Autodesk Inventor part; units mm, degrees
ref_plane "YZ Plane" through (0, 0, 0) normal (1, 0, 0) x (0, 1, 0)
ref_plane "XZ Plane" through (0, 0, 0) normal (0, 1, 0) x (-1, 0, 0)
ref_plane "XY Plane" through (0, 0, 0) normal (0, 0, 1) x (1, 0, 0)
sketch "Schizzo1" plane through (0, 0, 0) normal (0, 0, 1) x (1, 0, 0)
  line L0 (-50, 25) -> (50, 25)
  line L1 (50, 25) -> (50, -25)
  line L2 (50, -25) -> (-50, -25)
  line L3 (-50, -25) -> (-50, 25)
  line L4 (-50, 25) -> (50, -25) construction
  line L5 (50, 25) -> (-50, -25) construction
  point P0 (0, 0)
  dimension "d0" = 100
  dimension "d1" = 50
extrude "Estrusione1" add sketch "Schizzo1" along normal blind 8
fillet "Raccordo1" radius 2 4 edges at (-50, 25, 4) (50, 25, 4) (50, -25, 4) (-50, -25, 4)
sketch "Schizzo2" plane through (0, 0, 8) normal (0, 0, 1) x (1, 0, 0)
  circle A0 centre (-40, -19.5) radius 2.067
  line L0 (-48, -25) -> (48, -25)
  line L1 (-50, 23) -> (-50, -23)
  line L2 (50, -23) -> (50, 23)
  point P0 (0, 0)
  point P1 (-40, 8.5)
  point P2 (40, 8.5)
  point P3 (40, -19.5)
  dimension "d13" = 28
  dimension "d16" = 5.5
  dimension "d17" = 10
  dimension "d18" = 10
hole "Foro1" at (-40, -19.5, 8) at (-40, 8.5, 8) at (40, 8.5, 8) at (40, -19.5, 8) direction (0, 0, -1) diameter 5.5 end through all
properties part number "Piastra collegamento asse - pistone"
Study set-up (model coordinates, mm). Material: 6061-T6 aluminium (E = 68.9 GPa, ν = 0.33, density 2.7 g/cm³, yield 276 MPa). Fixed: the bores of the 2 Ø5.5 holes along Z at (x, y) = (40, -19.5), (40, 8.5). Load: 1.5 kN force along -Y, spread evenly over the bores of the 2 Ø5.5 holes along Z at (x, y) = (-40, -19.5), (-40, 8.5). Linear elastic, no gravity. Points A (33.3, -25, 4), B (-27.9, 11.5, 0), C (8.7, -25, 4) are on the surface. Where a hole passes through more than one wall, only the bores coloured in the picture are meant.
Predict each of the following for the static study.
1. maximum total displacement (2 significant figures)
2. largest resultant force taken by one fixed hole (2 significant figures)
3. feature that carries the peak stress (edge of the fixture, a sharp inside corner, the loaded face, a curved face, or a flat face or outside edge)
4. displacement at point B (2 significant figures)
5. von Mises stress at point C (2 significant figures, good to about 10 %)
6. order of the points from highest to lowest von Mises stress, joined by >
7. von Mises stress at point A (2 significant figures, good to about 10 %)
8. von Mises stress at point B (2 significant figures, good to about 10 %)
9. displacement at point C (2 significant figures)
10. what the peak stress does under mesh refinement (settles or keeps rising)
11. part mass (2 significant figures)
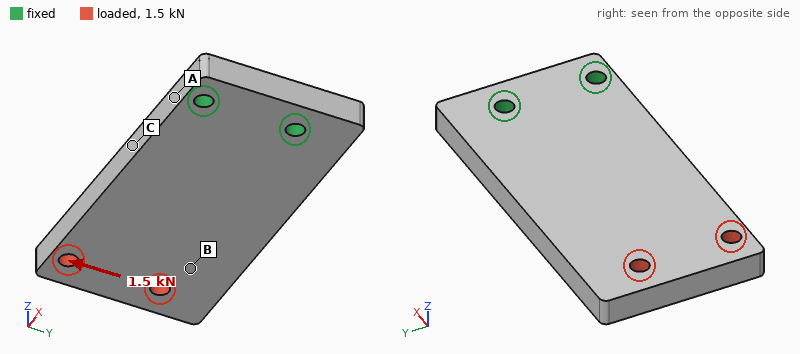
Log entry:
88 µm
4.0 kN
edge of the fixture
60 µm
23 MPa
A > C > B
39 MPa
8.1 MPa
26 µm
keeps rising
110 g
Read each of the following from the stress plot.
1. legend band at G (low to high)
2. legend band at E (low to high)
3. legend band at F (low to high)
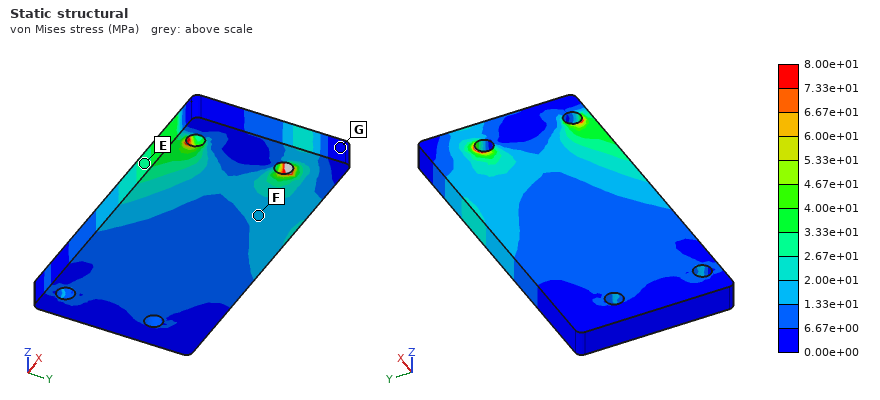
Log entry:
0.00e+00 to 6.67e+00 MPa
2.67e+01 to 3.33e+01 MPa
1.33e+01 to 2.00e+01 MPa
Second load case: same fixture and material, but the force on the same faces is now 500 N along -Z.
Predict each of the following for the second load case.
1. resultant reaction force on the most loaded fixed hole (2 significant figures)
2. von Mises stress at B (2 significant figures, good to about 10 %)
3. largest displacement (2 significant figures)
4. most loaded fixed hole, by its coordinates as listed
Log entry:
300 N
13 MPa
0.72 mm
(40, 8.5)
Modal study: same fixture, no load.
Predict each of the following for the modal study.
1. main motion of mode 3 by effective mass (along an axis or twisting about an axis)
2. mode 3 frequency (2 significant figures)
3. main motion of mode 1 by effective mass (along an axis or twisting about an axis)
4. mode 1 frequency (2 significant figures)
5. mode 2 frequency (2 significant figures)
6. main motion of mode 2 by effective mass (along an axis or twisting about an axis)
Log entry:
along Y
3700 Hz
along Z
810 Hz
3000 Hz
twisting about X
